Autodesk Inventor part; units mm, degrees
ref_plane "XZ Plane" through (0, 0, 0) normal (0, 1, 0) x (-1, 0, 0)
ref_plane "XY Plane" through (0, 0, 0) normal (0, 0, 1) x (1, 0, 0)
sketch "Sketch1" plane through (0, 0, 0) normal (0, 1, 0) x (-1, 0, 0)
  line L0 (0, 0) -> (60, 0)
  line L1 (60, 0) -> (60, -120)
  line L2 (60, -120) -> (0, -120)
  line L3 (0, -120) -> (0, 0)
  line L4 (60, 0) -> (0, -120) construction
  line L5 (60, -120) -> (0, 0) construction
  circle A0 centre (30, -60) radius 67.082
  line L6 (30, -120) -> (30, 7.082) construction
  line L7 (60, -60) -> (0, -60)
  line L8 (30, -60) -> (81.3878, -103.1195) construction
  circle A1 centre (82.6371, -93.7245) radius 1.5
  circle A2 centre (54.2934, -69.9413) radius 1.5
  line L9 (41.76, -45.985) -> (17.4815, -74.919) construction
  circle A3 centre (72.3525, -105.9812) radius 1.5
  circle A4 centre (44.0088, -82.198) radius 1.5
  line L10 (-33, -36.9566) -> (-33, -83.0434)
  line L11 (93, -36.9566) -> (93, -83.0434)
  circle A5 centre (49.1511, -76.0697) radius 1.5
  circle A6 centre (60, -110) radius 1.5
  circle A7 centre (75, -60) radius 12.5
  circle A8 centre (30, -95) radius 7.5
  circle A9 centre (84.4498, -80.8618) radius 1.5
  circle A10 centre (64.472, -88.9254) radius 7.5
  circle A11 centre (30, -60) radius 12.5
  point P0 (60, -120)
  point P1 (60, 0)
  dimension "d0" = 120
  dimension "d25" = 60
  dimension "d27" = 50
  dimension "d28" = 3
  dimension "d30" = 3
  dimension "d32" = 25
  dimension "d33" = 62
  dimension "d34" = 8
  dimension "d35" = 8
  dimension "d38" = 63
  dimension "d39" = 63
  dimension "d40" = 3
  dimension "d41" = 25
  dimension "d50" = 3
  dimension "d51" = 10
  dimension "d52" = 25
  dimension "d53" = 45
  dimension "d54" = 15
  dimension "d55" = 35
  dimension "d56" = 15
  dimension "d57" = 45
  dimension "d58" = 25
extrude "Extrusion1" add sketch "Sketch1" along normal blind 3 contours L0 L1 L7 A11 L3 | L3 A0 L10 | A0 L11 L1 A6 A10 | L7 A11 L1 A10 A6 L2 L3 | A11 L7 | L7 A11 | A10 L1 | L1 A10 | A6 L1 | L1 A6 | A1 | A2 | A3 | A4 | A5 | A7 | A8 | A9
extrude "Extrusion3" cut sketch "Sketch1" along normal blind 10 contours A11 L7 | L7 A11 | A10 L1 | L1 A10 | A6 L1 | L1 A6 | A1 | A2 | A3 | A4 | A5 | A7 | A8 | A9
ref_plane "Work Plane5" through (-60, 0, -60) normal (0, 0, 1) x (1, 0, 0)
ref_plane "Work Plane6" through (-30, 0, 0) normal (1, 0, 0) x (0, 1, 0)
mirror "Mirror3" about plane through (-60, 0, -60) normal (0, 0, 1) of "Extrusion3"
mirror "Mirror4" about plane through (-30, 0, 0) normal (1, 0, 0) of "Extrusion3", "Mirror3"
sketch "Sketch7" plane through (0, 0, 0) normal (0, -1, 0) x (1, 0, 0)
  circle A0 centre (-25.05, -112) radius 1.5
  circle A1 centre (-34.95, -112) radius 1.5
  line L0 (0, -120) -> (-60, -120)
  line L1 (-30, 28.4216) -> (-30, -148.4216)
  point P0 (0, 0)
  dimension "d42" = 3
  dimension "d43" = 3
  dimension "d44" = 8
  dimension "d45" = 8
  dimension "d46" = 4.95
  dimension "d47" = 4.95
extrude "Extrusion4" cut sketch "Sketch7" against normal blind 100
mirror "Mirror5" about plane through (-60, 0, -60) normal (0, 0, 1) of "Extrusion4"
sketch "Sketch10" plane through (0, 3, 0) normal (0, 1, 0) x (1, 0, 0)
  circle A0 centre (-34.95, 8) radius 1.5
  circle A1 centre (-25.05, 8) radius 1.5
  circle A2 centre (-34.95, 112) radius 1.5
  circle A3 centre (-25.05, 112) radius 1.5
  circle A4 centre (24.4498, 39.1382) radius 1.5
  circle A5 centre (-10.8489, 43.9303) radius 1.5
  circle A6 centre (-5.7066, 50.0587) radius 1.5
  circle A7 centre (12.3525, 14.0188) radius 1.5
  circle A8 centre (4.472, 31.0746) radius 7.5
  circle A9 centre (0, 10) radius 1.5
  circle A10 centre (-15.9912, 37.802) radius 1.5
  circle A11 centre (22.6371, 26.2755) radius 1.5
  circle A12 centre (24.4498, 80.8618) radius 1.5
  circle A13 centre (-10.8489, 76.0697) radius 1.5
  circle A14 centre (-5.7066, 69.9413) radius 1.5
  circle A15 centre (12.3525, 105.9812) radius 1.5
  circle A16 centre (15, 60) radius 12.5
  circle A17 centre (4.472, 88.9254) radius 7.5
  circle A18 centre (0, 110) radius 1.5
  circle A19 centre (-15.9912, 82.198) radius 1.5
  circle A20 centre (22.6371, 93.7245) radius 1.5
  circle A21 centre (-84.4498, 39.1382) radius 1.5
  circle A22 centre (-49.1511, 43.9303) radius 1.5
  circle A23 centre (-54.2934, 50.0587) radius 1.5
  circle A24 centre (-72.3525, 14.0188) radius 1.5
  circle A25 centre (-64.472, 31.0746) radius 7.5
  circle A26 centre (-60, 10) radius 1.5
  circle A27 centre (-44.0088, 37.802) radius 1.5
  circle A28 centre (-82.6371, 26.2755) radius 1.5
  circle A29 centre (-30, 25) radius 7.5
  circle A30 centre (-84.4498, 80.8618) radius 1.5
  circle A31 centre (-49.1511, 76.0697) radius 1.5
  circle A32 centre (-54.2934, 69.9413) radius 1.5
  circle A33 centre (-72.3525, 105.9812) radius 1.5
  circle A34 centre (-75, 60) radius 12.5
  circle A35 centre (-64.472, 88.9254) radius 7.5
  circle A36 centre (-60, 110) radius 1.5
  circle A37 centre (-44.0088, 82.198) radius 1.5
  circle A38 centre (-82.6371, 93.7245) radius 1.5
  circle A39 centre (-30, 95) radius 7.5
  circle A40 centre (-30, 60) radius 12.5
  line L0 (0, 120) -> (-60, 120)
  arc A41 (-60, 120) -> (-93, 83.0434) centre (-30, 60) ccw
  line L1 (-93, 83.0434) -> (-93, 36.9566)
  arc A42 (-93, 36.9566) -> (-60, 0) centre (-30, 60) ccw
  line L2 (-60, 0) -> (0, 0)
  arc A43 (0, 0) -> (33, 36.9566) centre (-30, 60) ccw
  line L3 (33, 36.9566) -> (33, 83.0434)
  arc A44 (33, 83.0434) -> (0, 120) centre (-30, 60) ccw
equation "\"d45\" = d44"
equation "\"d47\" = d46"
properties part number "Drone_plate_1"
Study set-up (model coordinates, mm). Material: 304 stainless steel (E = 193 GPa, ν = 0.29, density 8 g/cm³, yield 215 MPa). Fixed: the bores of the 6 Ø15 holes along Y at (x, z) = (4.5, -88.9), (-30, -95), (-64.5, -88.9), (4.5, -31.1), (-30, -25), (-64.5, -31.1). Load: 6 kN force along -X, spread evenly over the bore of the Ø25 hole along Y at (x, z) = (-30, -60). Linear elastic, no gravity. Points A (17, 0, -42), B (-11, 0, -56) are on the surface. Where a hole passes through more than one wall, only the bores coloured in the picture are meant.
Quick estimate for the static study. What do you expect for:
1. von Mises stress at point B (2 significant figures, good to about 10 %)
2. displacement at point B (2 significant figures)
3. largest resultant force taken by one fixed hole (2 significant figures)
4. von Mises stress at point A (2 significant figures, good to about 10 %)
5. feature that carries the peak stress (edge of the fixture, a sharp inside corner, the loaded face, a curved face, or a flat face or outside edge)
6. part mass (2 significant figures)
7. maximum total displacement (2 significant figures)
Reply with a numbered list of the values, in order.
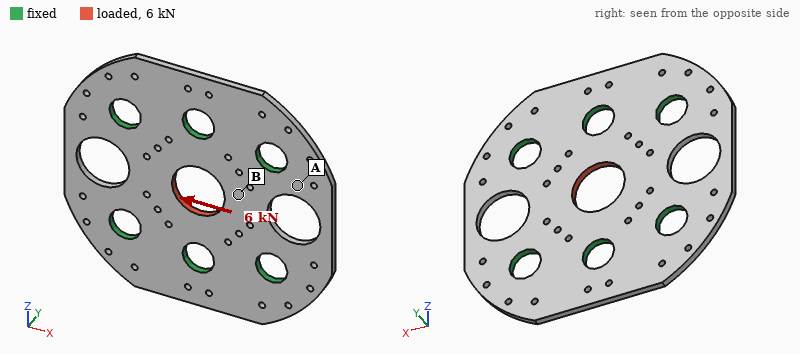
1. 20 MPa
2. 3.4 µm
3. 1.3 kN
4. 6.2 MPa
5. a curved face
6. 250 g
7. 4.3 µm
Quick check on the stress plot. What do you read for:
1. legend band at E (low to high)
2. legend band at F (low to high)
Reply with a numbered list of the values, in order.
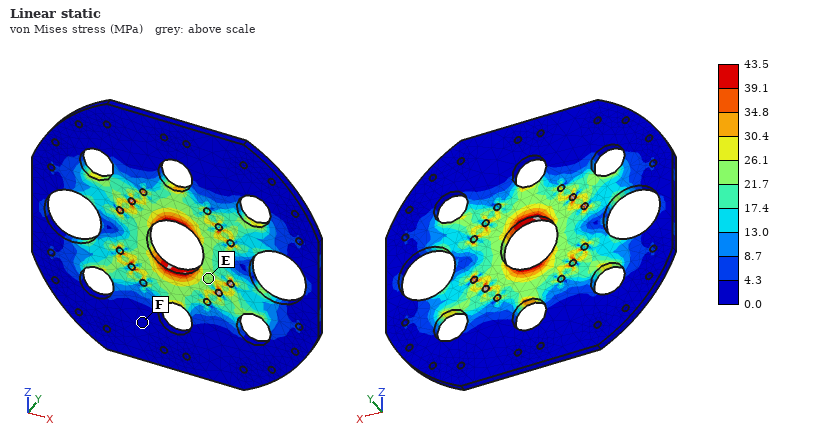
1. 21.7 to 26.1 MPa
2. 0.0 to 4.3 MPa
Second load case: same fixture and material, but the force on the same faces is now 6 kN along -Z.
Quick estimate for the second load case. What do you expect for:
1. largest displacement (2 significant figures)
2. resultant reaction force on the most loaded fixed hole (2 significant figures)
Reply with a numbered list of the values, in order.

1. 3.0 µm
2. 1.8 kN
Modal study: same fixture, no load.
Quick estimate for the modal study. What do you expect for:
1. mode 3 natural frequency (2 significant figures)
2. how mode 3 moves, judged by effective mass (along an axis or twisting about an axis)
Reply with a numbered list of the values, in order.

1. 5200 Hz
2. twisting about X
